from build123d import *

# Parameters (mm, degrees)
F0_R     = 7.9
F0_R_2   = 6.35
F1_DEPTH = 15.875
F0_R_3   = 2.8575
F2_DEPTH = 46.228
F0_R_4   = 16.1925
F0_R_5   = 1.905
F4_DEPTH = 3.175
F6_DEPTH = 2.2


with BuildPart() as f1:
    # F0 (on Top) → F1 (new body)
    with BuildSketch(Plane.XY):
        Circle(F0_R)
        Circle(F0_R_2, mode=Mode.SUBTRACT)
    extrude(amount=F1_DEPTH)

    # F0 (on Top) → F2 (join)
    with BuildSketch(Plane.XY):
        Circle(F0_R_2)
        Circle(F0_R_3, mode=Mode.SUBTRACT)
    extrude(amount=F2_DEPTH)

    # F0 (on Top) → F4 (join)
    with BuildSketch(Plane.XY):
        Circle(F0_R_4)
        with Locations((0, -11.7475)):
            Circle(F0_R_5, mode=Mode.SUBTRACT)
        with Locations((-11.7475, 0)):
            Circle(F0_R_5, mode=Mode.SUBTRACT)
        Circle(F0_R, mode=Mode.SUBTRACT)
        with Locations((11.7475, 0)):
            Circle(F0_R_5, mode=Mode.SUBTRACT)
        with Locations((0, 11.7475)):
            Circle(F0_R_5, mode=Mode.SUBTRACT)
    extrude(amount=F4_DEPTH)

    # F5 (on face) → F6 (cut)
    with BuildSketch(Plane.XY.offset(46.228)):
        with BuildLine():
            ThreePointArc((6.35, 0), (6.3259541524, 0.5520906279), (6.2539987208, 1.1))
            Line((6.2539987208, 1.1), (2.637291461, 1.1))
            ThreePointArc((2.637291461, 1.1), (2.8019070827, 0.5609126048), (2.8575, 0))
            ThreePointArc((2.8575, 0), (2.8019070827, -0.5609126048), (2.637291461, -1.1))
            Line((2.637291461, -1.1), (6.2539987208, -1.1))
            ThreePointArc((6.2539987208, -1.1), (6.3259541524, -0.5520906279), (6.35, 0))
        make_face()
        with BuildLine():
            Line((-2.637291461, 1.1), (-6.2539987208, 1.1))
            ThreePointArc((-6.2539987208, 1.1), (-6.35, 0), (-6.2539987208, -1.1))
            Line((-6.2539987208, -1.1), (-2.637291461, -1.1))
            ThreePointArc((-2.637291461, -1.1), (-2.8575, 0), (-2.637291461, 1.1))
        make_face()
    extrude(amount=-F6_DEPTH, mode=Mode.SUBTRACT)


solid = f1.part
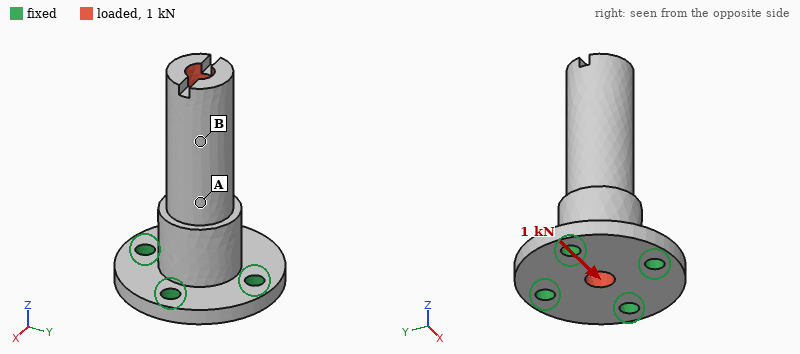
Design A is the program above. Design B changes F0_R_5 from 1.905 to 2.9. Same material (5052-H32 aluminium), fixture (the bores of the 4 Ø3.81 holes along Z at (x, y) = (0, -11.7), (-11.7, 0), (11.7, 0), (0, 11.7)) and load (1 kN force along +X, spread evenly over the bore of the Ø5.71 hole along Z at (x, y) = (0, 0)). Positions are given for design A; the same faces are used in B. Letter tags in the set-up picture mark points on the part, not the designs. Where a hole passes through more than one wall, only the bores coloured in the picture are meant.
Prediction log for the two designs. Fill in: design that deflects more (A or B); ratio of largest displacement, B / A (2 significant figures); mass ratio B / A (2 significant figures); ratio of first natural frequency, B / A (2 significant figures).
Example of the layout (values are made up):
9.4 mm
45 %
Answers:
A
0.86
0.97
1.1
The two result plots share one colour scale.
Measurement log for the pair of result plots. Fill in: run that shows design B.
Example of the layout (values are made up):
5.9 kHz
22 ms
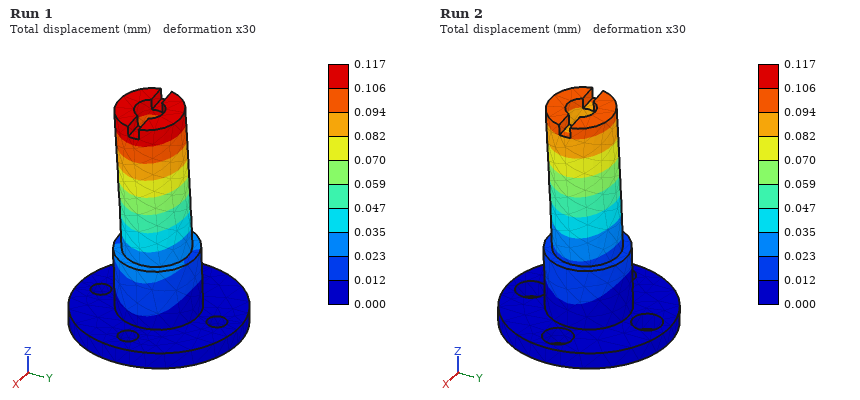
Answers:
Run 2
